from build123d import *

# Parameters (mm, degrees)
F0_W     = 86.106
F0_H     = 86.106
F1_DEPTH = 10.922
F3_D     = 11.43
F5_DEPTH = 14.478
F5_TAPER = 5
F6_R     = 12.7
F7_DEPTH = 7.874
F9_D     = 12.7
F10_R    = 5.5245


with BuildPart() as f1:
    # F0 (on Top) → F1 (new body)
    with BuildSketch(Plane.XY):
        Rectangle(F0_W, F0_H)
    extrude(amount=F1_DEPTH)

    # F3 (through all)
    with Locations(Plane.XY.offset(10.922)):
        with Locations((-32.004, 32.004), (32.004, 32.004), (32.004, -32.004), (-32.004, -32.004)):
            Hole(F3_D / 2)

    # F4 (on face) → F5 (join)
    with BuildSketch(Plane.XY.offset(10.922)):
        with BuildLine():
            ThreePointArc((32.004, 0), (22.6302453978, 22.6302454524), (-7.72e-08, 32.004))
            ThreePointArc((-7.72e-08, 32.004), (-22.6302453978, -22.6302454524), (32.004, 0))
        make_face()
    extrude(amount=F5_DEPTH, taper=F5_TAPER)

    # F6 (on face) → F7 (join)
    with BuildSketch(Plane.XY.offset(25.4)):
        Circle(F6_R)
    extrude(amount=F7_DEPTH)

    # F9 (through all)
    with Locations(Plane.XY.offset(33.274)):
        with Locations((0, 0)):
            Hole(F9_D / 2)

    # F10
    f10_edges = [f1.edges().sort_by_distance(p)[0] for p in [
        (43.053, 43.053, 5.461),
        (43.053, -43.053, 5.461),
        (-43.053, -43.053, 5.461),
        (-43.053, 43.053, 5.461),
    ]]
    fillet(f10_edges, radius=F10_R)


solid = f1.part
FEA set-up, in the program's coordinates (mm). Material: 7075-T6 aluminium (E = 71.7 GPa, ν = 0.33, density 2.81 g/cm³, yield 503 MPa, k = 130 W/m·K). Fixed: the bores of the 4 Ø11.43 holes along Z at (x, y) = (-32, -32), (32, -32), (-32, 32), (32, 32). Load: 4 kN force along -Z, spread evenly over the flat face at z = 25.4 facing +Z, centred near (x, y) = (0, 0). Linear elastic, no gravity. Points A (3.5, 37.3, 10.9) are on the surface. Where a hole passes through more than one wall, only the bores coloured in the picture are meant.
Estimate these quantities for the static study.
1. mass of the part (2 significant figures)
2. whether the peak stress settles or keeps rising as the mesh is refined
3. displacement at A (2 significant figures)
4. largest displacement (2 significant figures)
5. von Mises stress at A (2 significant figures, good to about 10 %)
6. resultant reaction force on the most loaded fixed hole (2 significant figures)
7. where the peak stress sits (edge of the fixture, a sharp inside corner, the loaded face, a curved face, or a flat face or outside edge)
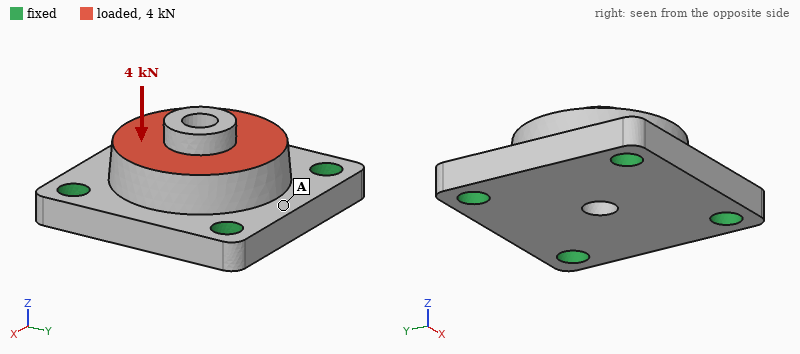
340 g
keeps rising
2.8 µm
4.2 µm
3.1 MPa
1.1 kN
edge of the fixture
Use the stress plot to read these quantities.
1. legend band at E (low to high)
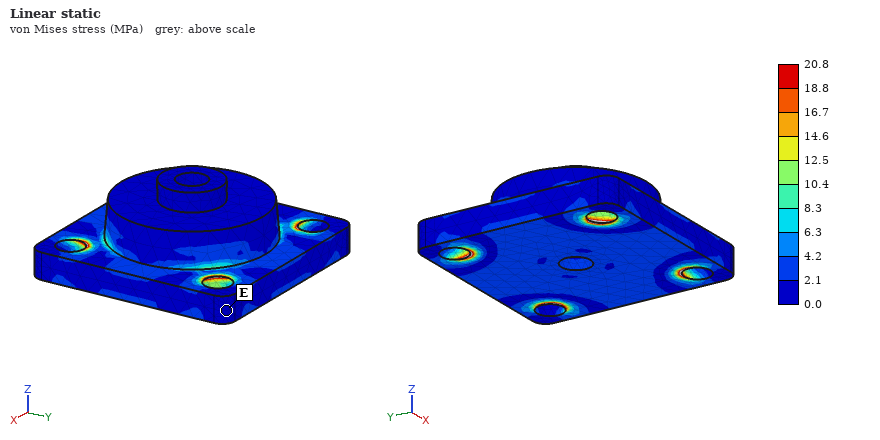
0.0 to 2.1 MPa
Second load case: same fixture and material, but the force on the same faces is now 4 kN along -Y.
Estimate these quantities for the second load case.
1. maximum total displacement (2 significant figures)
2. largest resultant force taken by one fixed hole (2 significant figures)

5.0 µm
1.3 kN
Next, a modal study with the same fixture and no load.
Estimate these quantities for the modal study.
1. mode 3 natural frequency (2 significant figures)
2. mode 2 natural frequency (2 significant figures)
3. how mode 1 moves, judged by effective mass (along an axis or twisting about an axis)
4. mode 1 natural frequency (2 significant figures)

13 kHz
13 kHz
along Z
10 kHz
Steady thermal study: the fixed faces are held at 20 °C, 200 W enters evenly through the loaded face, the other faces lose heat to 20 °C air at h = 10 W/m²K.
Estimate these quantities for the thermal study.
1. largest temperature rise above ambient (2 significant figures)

26 K
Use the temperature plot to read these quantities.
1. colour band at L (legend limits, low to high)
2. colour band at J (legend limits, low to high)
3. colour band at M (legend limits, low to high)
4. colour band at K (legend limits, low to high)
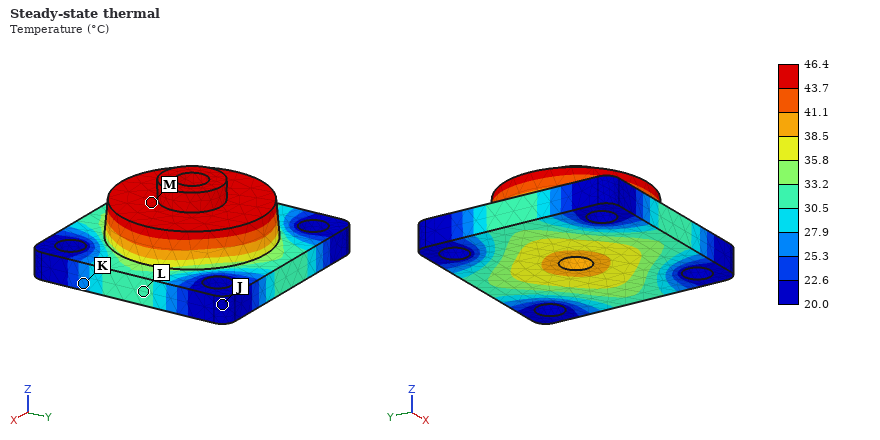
30.5 to 33.2 °C
20.0 to 22.6 °C
43.7 to 46.4 °C
25.3 to 27.9 °C
